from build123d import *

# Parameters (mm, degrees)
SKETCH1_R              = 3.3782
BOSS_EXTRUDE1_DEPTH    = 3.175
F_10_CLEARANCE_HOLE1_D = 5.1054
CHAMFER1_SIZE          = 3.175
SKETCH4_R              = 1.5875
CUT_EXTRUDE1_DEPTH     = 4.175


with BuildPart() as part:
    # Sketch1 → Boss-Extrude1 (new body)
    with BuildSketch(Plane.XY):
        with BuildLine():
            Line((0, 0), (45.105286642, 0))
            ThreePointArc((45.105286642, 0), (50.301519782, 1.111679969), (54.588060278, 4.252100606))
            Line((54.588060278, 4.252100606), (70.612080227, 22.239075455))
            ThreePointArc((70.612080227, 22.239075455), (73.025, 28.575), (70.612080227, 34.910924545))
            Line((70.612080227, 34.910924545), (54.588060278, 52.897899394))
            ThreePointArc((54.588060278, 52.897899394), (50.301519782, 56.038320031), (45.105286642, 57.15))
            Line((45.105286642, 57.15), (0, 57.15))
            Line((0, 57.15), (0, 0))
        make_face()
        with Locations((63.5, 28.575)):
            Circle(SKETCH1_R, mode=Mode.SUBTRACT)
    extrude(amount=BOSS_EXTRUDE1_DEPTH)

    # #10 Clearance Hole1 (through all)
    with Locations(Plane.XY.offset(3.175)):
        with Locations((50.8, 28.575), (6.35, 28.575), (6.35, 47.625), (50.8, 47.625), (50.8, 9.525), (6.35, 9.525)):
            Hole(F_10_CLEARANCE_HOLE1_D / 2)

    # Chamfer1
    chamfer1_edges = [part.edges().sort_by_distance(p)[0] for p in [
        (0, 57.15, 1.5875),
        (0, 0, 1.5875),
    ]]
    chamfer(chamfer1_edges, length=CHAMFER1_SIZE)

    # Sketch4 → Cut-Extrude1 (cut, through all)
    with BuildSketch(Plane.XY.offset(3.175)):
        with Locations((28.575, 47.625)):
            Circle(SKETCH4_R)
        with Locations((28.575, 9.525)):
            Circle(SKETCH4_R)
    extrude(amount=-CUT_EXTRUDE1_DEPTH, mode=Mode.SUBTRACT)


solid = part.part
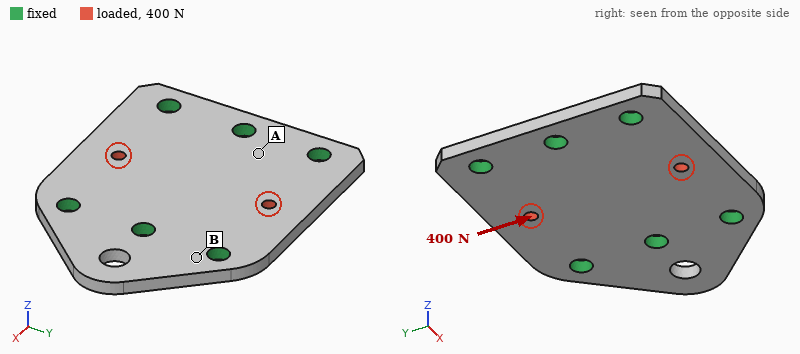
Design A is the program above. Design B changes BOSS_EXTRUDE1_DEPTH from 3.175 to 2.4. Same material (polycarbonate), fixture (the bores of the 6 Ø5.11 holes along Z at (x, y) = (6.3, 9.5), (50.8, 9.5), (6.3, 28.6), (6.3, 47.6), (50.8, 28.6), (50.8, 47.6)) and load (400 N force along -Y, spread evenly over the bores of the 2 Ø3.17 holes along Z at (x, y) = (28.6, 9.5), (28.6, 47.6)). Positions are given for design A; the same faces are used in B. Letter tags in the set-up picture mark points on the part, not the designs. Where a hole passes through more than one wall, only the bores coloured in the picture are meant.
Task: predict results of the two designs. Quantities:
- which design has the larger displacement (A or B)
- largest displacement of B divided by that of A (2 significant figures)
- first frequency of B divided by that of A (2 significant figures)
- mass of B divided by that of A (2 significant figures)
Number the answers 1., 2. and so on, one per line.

1. B
2. 1.3
3. 0.78
4. 0.76
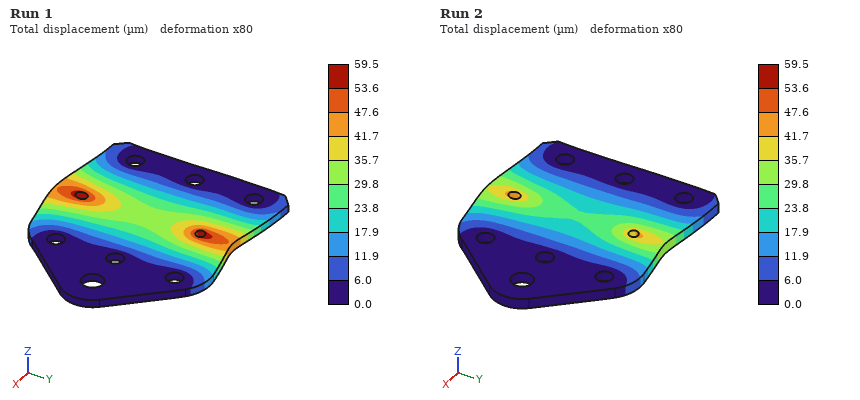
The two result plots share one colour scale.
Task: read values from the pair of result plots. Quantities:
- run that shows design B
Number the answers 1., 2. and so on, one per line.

1. Run 1
